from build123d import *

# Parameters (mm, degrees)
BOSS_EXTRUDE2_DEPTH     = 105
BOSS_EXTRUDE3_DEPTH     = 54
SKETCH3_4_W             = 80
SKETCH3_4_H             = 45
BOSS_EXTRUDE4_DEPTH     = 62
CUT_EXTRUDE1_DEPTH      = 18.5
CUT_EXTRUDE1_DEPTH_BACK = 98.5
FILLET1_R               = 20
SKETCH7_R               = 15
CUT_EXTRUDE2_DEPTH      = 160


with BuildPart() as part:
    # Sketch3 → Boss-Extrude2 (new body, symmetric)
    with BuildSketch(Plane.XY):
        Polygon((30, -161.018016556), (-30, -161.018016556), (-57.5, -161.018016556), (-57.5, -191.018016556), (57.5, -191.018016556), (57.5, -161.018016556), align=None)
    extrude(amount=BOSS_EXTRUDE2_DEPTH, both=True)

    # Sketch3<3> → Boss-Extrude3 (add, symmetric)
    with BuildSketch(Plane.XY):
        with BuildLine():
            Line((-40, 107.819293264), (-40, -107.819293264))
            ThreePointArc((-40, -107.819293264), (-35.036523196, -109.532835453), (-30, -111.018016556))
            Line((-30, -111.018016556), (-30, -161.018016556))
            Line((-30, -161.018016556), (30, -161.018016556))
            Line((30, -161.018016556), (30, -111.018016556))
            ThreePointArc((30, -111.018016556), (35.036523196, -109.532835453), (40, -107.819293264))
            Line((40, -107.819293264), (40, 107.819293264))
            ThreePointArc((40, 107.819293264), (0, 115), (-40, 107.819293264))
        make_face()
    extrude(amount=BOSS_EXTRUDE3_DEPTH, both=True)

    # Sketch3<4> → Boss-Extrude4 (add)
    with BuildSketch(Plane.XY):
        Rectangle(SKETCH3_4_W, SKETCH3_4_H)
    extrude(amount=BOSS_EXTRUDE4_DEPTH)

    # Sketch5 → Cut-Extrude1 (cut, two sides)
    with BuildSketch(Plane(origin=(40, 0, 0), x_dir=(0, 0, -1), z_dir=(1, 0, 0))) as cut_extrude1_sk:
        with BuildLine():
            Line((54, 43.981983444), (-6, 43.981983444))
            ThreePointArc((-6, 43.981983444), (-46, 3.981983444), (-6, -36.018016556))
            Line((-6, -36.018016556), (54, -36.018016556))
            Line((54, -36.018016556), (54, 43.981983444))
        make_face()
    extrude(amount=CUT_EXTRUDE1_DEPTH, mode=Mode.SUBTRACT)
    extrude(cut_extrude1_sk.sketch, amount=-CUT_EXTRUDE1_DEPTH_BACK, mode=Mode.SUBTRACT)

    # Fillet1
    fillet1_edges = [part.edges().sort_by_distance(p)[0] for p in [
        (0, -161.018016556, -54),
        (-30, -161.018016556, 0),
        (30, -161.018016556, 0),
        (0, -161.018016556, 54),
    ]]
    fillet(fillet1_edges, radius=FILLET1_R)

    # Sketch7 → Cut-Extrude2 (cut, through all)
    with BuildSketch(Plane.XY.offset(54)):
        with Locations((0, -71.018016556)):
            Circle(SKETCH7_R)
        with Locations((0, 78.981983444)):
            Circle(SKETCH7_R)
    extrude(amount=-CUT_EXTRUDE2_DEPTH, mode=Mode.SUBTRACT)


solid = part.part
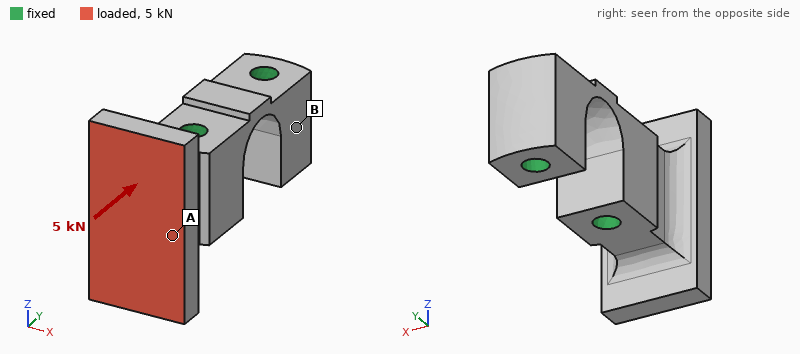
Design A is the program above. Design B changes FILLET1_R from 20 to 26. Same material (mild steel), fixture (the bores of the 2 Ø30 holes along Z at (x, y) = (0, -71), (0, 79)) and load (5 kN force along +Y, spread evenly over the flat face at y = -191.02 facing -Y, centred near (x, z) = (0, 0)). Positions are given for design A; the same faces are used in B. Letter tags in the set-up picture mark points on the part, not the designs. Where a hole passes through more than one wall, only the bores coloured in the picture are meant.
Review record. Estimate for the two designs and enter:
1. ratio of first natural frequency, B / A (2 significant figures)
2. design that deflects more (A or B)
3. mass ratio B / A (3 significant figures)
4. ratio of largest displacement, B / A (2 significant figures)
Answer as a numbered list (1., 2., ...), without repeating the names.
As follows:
1. 1.00
2. A
3. 1.01
4. 0.88
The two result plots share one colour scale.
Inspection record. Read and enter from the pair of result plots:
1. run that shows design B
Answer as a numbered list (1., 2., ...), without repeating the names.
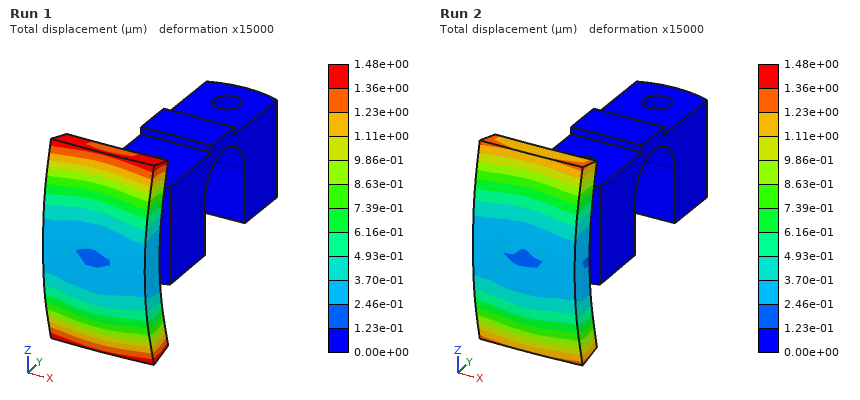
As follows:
1. Run 2
